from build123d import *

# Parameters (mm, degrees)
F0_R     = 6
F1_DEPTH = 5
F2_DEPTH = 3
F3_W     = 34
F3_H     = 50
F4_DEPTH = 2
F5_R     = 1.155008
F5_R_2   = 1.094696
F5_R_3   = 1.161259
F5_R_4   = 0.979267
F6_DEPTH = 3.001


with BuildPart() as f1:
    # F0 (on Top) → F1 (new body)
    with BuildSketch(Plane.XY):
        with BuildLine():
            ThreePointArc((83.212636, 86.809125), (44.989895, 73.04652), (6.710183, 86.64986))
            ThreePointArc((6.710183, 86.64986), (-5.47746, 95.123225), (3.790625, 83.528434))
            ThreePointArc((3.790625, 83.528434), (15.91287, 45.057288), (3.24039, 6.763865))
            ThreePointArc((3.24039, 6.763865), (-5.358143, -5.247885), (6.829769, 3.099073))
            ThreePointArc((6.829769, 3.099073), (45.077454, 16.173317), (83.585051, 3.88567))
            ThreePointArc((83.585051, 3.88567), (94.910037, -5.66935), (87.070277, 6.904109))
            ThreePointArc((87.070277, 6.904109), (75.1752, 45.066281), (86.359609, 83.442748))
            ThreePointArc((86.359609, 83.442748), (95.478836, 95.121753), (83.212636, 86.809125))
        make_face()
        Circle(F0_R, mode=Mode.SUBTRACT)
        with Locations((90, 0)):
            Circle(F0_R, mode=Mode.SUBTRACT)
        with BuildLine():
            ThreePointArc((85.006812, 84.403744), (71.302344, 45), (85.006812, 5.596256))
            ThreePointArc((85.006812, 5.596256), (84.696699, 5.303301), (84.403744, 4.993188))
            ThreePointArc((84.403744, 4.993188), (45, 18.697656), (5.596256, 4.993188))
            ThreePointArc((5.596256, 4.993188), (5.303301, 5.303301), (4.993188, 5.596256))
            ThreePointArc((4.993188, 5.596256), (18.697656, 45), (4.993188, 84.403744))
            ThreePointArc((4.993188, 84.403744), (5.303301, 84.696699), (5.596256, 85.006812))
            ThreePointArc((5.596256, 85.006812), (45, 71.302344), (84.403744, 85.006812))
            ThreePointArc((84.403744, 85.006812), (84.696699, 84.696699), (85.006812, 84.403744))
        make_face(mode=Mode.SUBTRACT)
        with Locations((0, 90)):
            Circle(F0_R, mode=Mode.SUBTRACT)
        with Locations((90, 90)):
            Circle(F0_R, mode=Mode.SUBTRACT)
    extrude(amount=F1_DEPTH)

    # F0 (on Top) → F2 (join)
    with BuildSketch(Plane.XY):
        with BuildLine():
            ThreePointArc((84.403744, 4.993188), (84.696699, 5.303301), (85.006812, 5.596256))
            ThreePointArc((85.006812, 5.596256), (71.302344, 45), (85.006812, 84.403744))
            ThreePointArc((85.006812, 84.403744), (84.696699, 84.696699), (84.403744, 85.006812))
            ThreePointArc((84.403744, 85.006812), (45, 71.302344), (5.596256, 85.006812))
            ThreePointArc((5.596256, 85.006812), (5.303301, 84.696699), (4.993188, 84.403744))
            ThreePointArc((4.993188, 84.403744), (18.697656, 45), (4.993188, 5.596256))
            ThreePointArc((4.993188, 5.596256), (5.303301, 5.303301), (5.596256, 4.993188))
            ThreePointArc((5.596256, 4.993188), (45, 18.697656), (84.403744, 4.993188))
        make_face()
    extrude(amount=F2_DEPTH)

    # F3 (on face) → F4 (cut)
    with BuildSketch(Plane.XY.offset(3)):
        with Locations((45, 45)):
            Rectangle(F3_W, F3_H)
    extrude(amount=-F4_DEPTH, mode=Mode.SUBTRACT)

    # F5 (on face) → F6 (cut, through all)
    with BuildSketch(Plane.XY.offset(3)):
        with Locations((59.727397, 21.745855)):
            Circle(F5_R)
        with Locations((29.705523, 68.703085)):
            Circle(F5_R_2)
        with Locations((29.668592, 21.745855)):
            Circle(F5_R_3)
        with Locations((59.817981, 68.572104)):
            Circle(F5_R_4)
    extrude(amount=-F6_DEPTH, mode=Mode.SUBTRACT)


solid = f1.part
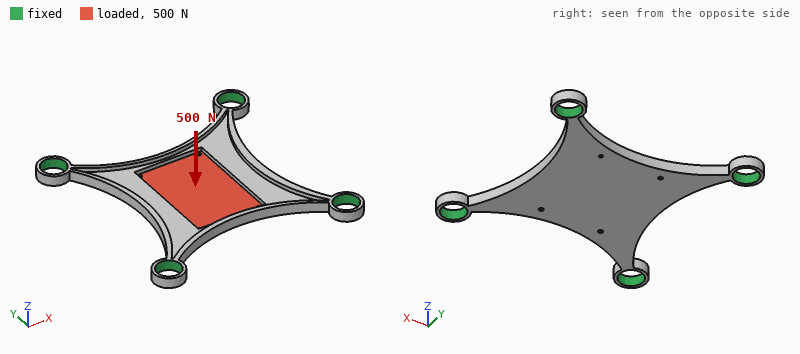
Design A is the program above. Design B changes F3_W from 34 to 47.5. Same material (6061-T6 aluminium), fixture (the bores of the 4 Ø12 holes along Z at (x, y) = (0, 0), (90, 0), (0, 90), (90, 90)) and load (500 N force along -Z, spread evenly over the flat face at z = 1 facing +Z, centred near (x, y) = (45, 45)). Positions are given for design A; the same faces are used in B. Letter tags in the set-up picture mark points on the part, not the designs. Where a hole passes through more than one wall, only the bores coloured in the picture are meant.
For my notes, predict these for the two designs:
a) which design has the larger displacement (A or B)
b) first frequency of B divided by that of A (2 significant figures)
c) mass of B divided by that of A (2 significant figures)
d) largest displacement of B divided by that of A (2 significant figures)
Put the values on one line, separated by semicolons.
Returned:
B; 1.0; 0.89; 1.2
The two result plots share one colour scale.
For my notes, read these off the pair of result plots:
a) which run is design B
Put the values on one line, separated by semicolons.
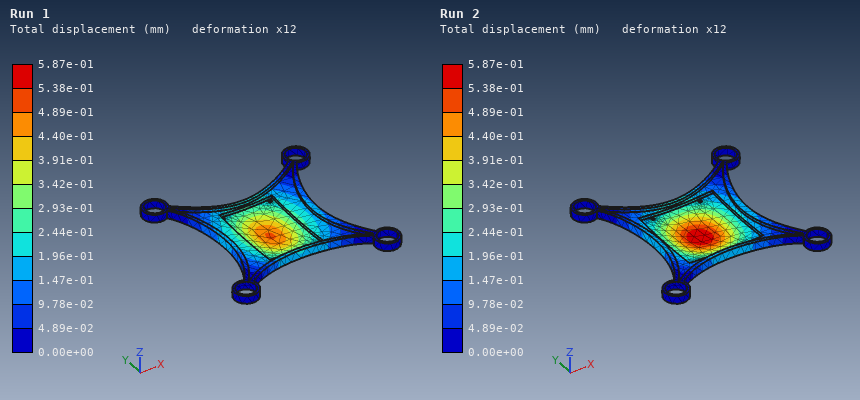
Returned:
Run 2
